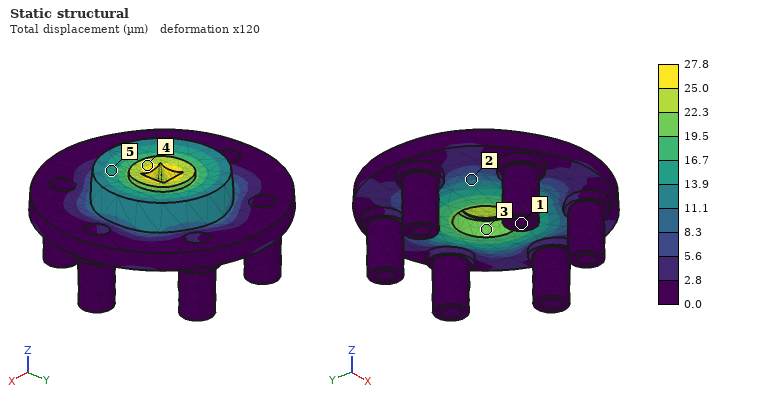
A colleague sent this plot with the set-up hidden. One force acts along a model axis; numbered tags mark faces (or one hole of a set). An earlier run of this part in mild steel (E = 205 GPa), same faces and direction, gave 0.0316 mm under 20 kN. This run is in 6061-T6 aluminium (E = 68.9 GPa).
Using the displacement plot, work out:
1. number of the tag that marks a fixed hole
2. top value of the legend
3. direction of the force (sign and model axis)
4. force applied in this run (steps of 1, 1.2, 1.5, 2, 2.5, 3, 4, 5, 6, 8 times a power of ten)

1
27.8 µm
-Z
6 kN
